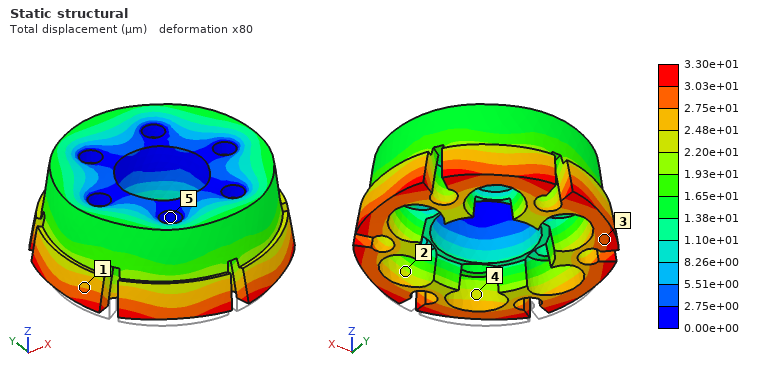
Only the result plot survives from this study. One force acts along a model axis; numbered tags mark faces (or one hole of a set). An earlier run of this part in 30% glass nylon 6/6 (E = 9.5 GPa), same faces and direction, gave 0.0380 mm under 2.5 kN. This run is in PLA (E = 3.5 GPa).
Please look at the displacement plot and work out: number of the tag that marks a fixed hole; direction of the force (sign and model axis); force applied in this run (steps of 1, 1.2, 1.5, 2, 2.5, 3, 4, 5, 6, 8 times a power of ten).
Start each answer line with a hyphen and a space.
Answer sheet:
- 5
- +Z
- 800 N
